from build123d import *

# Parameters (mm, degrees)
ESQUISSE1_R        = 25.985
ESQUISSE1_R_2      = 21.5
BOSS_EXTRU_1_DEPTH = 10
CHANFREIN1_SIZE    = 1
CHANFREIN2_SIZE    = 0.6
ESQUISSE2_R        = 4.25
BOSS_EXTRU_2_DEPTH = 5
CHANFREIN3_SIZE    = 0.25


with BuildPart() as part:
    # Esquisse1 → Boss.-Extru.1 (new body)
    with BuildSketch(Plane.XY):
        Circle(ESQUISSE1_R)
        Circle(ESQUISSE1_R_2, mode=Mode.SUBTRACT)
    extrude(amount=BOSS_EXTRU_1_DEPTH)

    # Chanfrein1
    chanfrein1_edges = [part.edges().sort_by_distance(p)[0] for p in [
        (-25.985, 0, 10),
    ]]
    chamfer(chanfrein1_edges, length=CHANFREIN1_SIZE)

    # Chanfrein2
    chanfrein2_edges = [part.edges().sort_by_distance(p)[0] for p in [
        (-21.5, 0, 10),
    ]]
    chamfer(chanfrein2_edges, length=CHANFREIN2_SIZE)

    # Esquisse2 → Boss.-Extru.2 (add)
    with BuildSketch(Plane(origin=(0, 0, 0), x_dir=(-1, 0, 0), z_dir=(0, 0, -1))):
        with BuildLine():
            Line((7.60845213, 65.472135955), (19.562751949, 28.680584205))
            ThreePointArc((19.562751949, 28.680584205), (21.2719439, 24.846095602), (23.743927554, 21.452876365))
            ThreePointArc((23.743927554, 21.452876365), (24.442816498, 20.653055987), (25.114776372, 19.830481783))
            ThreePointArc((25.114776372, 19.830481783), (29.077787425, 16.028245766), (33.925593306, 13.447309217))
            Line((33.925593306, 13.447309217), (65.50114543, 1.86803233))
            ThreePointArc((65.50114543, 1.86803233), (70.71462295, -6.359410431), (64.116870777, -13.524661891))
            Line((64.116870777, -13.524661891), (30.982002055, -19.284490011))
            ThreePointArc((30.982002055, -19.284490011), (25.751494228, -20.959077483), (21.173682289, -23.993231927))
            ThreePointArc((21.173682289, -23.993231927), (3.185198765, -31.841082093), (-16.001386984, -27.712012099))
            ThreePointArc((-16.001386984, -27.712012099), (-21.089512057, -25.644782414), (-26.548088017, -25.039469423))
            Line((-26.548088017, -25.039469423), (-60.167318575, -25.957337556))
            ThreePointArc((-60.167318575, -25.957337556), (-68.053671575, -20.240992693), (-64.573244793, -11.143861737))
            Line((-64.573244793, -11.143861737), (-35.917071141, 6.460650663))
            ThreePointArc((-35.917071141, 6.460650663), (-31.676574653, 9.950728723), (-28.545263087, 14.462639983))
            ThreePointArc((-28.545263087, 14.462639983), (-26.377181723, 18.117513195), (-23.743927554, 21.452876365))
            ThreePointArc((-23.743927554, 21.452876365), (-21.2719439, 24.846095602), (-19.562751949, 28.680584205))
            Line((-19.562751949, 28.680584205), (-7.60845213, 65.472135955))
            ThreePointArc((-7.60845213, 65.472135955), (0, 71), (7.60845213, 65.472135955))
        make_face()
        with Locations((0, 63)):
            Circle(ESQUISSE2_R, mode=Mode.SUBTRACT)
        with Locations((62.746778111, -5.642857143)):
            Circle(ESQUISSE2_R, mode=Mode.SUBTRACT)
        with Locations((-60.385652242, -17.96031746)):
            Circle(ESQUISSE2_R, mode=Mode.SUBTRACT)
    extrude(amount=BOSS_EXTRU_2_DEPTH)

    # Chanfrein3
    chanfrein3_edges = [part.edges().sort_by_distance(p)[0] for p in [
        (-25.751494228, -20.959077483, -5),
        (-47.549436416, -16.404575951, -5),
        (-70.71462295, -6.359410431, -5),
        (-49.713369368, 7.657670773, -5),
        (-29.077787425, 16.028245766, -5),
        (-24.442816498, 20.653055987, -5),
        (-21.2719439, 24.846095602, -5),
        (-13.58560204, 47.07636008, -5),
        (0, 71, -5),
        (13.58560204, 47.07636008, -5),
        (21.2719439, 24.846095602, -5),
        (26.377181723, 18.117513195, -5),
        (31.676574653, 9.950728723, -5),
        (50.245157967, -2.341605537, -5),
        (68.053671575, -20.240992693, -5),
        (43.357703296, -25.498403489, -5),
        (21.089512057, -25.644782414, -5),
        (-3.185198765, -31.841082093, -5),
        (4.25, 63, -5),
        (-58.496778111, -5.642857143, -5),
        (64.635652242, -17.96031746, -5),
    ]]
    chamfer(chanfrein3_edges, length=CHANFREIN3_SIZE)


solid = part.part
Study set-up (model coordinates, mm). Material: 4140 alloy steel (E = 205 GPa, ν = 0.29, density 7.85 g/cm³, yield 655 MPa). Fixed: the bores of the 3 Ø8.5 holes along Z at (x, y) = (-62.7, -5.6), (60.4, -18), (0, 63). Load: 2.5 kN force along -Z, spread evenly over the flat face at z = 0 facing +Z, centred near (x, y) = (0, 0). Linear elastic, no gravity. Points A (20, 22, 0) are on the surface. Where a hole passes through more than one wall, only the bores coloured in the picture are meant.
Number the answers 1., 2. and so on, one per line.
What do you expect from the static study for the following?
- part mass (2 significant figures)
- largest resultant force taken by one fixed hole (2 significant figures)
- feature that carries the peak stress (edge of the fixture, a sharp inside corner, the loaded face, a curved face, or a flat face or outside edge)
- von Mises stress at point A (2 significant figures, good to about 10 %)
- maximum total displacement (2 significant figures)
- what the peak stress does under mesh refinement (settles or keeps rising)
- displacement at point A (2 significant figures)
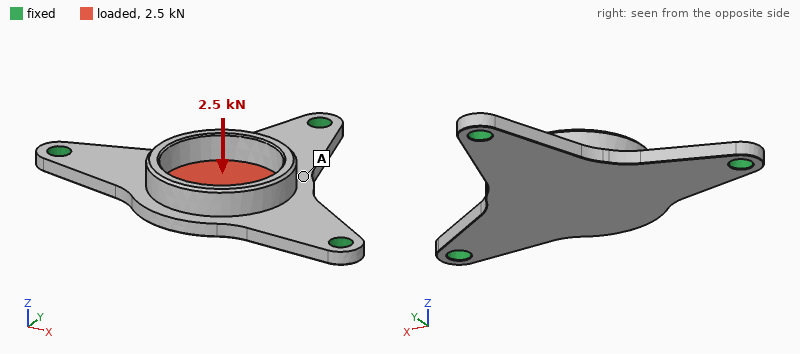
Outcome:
1. 280 g
2. 1.1 kN
3. edge of the fixture
4. 26 MPa
5. 0.16 mm
6. keeps rising
7. 0.071 mm
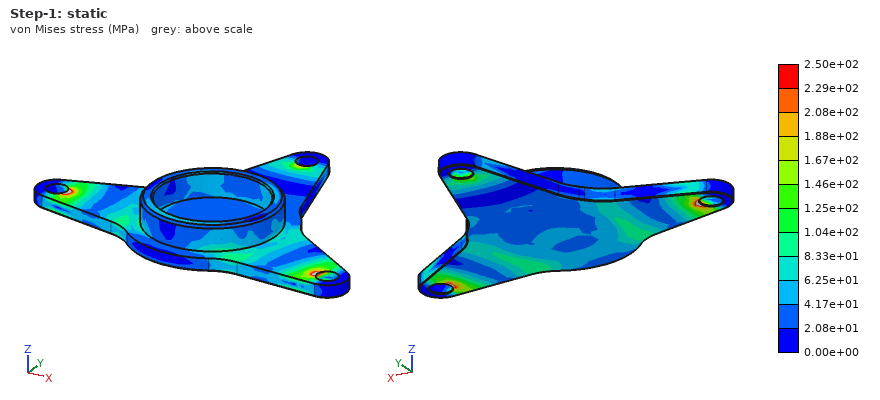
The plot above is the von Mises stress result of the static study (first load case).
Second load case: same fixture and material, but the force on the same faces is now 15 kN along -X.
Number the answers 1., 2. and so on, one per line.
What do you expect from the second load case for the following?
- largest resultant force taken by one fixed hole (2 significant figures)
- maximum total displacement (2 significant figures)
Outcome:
1. 7.3 kN
2. 32 µm
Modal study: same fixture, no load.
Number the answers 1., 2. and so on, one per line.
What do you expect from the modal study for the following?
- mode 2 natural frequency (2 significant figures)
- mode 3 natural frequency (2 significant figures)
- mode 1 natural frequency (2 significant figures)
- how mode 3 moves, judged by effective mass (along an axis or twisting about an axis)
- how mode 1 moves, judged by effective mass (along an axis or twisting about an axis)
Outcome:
1. 3300 Hz
2. 4100 Hz
3. 1700 Hz
4. twisting about Y
5. along Z
